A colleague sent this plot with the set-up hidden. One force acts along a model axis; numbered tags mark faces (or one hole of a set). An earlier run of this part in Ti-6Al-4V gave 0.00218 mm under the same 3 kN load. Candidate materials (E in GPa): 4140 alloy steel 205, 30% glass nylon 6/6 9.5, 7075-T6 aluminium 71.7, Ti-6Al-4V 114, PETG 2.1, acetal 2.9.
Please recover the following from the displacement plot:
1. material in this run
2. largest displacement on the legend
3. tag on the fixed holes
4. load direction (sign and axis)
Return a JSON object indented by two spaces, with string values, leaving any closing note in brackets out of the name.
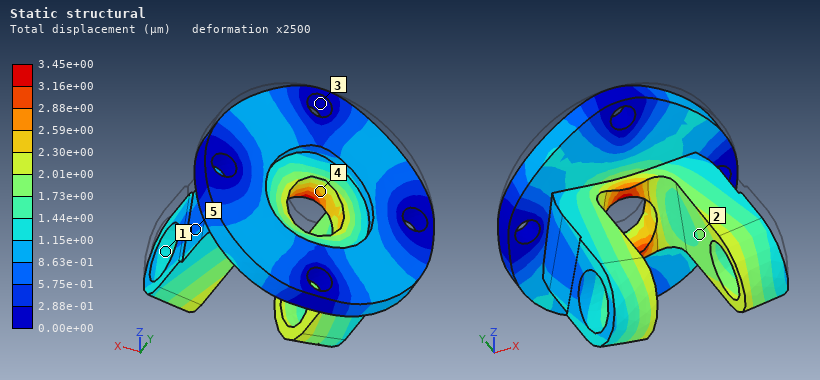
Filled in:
{
  "material in this run": "7075-T6 aluminium",
  "largest displacement on the legend": "3.45e+00 µm",
  "tag on the fixed holes": "3",
  "load direction": "-Z"
}
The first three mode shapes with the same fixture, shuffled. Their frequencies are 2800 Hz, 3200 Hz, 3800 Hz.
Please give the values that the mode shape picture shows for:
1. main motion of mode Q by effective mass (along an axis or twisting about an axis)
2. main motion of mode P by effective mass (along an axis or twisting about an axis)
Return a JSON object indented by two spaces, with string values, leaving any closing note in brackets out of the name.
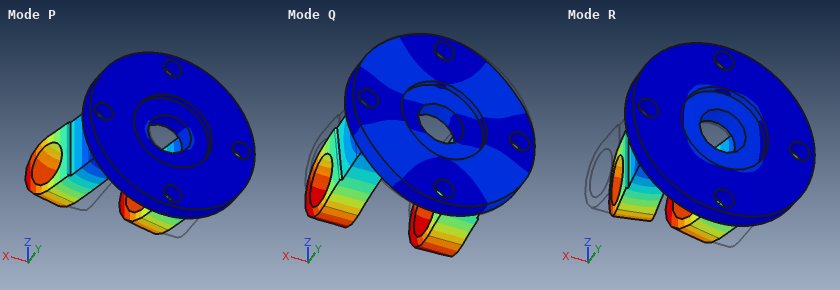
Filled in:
{
  "main motion of mode Q by effective mass": "along Z",
  "main motion of mode P by effective mass": "along X"
}
